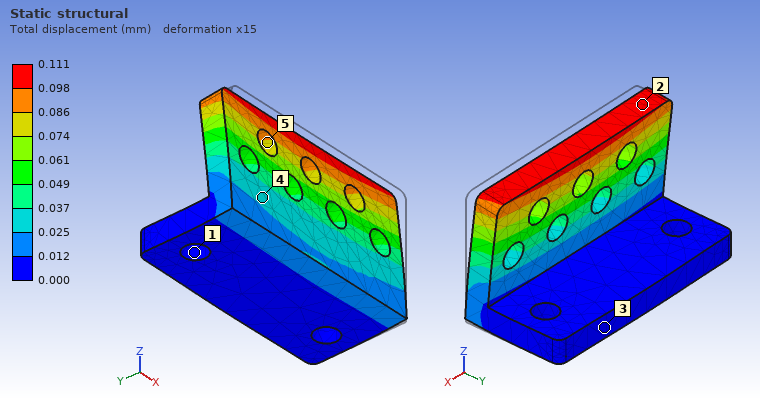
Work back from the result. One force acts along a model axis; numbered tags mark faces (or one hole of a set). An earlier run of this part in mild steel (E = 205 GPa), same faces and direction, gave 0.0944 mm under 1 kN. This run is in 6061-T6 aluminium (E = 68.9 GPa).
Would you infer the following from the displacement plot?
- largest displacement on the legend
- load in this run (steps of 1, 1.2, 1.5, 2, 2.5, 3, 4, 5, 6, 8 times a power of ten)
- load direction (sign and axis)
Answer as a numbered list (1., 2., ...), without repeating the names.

1. 0.111 mm
2. 400 N
3. +Y
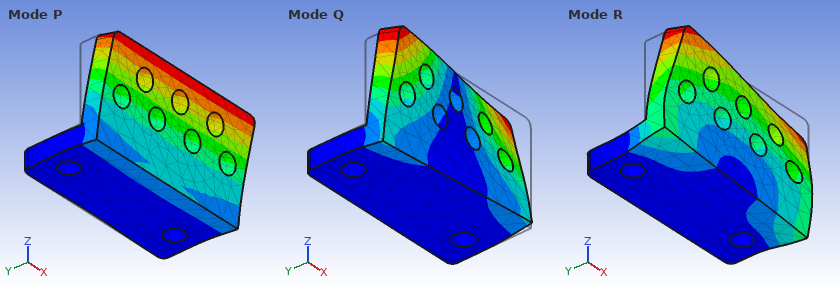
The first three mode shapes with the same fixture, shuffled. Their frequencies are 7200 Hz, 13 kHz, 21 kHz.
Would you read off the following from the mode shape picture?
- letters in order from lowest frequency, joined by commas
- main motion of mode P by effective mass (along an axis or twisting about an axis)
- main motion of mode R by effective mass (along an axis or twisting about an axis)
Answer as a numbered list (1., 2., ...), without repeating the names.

1. P, Q, R
2. along Y
3. along X
